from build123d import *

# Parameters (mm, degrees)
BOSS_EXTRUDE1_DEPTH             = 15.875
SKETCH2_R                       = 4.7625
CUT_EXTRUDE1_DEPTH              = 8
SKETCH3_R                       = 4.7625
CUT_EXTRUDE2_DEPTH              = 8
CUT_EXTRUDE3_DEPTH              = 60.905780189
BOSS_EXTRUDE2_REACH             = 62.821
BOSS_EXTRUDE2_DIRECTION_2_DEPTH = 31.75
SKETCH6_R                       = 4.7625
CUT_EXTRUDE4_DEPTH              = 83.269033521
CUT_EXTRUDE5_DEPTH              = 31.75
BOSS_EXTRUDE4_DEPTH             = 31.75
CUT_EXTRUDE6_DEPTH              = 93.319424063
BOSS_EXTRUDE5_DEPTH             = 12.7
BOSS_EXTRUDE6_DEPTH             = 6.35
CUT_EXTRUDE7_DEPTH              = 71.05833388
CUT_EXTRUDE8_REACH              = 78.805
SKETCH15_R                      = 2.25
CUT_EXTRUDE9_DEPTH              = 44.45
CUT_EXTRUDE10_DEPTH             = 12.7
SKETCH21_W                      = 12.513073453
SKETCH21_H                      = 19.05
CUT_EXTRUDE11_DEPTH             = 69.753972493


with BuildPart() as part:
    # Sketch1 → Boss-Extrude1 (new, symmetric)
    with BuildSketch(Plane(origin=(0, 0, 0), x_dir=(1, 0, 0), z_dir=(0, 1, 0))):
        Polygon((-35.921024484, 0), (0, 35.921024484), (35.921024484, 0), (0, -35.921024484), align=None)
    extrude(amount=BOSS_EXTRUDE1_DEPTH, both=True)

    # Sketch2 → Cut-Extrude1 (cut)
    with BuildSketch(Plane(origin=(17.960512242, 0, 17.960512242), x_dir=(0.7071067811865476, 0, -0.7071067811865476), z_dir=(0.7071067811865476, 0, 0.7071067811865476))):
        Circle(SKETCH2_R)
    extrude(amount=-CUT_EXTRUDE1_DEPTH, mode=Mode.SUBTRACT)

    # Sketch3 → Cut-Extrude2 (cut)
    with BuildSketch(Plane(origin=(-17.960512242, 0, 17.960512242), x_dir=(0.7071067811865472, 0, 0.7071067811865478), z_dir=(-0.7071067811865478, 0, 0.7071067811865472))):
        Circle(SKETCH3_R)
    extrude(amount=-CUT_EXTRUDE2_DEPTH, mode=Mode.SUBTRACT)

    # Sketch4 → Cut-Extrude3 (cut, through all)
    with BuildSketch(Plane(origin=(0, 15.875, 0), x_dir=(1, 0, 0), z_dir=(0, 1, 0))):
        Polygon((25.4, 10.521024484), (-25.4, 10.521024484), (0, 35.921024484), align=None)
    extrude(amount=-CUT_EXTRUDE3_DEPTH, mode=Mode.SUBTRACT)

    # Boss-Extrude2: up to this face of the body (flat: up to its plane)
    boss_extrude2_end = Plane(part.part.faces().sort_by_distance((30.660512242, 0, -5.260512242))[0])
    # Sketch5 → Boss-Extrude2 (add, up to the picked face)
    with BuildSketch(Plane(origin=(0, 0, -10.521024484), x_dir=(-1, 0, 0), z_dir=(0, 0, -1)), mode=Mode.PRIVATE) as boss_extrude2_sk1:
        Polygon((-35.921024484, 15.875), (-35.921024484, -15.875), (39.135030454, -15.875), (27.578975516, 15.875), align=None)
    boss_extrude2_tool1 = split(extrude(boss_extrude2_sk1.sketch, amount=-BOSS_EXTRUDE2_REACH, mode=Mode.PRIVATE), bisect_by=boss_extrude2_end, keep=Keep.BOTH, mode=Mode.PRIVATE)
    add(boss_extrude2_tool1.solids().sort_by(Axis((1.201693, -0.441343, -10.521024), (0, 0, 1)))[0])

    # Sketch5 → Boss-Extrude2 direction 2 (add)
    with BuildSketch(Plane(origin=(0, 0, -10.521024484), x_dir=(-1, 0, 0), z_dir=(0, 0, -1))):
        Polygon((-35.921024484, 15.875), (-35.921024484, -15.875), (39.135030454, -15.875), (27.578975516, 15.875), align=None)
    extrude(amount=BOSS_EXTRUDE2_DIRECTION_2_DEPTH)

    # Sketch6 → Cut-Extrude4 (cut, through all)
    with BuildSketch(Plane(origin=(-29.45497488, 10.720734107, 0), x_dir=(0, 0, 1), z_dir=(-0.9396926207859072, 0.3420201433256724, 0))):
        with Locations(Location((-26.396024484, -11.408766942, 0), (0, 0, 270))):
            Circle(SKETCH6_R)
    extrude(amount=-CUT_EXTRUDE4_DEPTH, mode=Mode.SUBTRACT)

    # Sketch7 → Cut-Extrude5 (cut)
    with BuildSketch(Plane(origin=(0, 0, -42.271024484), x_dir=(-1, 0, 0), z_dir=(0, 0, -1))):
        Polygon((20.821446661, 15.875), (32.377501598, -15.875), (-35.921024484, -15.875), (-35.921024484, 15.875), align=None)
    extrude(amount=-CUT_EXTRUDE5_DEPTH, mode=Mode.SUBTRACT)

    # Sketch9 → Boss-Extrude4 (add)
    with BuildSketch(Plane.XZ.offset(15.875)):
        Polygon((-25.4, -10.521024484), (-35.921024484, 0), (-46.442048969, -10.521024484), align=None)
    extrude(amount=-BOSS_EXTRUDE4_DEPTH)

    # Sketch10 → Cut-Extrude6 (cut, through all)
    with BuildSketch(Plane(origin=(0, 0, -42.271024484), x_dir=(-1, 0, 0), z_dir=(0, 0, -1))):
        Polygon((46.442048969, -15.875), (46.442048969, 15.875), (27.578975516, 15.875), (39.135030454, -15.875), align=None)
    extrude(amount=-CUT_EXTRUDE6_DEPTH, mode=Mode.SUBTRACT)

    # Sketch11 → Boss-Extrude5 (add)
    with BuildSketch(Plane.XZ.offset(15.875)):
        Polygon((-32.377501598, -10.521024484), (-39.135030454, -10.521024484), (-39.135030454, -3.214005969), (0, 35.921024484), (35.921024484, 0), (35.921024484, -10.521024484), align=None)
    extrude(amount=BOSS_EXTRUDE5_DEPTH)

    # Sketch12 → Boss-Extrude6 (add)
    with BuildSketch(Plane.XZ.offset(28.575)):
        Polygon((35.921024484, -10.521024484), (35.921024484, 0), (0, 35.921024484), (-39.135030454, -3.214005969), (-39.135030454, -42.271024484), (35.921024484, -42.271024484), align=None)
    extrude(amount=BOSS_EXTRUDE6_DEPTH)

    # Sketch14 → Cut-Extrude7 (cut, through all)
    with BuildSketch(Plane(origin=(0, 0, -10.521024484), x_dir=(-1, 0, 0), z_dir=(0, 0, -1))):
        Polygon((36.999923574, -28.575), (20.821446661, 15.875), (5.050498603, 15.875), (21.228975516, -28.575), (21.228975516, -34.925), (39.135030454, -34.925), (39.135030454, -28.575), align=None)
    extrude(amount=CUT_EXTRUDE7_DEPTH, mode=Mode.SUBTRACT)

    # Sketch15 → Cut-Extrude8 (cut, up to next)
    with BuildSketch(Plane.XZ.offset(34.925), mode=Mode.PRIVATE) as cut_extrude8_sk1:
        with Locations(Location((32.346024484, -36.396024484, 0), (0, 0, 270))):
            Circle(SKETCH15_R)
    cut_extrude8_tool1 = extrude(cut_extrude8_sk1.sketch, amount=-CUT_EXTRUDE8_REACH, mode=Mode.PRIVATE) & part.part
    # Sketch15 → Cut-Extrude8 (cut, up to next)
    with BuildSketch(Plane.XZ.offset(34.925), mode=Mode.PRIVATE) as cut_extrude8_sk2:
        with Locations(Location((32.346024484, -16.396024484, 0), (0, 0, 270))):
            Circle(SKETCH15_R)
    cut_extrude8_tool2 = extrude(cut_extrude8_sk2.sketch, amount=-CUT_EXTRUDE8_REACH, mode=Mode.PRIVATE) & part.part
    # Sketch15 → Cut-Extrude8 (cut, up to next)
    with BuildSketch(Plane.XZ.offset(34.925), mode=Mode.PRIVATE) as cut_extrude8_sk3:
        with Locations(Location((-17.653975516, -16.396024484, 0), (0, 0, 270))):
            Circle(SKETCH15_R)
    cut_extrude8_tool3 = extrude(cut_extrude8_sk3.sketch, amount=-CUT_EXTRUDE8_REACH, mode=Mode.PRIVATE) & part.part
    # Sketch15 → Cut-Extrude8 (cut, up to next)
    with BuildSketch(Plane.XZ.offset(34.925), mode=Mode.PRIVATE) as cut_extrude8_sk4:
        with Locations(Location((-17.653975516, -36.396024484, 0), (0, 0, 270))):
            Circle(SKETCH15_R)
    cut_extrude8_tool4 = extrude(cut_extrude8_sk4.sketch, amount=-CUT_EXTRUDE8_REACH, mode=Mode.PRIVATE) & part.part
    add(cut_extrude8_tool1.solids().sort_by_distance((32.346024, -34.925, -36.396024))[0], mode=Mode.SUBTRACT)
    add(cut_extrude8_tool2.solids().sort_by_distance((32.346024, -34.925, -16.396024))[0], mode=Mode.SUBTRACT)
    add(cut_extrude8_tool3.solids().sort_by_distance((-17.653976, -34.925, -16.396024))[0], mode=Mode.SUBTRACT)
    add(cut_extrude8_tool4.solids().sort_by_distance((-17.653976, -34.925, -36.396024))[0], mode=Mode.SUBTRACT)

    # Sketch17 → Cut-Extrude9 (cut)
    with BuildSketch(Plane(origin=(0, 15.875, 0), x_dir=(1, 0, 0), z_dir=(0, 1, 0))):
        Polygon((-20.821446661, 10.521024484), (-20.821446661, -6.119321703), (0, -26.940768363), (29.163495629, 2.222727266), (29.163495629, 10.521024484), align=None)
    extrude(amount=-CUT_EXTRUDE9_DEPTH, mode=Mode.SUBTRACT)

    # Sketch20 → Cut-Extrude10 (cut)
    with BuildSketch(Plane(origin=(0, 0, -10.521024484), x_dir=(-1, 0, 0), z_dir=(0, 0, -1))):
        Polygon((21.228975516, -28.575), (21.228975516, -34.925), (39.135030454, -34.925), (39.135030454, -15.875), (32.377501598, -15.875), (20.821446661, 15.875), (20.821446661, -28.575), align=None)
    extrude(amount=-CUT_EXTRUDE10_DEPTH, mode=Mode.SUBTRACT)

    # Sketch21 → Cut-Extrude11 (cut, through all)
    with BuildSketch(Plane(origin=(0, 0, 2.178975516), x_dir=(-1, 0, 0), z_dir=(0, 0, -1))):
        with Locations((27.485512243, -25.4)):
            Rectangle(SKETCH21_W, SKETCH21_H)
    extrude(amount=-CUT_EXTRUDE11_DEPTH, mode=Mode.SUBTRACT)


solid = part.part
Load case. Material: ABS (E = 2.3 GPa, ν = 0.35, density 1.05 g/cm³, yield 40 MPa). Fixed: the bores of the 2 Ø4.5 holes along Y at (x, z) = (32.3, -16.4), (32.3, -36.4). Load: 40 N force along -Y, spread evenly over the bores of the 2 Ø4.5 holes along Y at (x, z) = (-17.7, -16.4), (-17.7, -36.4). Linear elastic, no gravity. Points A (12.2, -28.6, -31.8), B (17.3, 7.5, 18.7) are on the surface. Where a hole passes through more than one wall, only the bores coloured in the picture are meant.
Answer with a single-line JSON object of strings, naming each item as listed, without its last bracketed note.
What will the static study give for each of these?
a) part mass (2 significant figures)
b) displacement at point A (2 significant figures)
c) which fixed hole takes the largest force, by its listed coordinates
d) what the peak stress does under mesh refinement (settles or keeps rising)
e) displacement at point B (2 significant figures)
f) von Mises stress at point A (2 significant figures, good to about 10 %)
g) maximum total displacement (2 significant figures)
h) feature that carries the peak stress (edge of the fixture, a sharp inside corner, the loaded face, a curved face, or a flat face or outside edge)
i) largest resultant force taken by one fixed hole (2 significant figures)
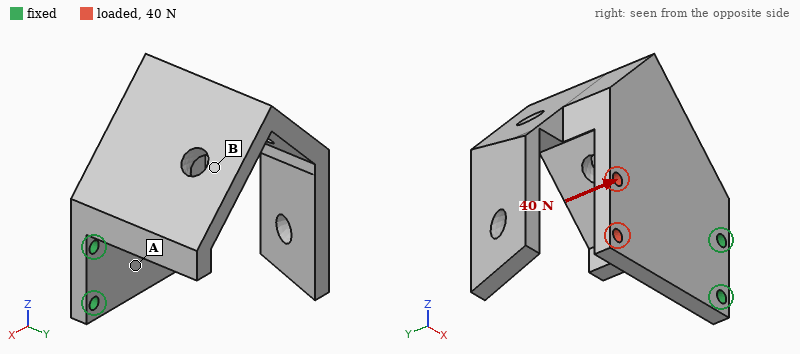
{"part mass": "60 g", "displacement at point A": "0.18 mm", "which fixed hole takes the largest force, by its listed coordinates": "(32.3, -16.4)", "what the peak stress does under mesh refinement": "keeps rising", "displacement at point B": "0.47 mm", "von Mises stress at point A": "3.3 MPa", "maximum total displacement": "1.0 mm", "feature that carries the peak stress": "edge of the fixture", "largest resultant force taken by one fixed hole": "24 N"}
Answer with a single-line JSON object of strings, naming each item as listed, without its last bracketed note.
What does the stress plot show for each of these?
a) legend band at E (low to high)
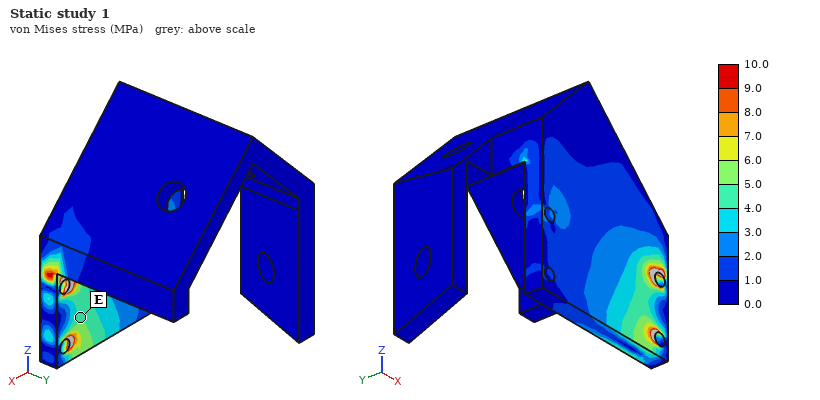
{"legend band at E": "4.0 to 5.0 MPa"}
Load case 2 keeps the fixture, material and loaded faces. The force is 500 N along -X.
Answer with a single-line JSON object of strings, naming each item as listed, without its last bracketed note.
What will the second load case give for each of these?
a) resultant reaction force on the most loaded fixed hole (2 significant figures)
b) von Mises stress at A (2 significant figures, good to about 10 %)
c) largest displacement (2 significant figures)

{"resultant reaction force on the most loaded fixed hole": "250 N", "von Mises stress at A": "2.5 MPa", "largest displacement": "87 µm"}
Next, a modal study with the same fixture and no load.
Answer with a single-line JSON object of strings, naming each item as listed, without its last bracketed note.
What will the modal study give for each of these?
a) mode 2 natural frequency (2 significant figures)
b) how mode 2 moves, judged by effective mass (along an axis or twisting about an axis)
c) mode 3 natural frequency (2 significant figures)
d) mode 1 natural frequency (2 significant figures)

{"mode 2 natural frequency": "200 Hz", "how mode 2 moves, judged by effective mass": "along Z", "mode 3 natural frequency": "260 Hz", "mode 1 natural frequency": "160 Hz"}
